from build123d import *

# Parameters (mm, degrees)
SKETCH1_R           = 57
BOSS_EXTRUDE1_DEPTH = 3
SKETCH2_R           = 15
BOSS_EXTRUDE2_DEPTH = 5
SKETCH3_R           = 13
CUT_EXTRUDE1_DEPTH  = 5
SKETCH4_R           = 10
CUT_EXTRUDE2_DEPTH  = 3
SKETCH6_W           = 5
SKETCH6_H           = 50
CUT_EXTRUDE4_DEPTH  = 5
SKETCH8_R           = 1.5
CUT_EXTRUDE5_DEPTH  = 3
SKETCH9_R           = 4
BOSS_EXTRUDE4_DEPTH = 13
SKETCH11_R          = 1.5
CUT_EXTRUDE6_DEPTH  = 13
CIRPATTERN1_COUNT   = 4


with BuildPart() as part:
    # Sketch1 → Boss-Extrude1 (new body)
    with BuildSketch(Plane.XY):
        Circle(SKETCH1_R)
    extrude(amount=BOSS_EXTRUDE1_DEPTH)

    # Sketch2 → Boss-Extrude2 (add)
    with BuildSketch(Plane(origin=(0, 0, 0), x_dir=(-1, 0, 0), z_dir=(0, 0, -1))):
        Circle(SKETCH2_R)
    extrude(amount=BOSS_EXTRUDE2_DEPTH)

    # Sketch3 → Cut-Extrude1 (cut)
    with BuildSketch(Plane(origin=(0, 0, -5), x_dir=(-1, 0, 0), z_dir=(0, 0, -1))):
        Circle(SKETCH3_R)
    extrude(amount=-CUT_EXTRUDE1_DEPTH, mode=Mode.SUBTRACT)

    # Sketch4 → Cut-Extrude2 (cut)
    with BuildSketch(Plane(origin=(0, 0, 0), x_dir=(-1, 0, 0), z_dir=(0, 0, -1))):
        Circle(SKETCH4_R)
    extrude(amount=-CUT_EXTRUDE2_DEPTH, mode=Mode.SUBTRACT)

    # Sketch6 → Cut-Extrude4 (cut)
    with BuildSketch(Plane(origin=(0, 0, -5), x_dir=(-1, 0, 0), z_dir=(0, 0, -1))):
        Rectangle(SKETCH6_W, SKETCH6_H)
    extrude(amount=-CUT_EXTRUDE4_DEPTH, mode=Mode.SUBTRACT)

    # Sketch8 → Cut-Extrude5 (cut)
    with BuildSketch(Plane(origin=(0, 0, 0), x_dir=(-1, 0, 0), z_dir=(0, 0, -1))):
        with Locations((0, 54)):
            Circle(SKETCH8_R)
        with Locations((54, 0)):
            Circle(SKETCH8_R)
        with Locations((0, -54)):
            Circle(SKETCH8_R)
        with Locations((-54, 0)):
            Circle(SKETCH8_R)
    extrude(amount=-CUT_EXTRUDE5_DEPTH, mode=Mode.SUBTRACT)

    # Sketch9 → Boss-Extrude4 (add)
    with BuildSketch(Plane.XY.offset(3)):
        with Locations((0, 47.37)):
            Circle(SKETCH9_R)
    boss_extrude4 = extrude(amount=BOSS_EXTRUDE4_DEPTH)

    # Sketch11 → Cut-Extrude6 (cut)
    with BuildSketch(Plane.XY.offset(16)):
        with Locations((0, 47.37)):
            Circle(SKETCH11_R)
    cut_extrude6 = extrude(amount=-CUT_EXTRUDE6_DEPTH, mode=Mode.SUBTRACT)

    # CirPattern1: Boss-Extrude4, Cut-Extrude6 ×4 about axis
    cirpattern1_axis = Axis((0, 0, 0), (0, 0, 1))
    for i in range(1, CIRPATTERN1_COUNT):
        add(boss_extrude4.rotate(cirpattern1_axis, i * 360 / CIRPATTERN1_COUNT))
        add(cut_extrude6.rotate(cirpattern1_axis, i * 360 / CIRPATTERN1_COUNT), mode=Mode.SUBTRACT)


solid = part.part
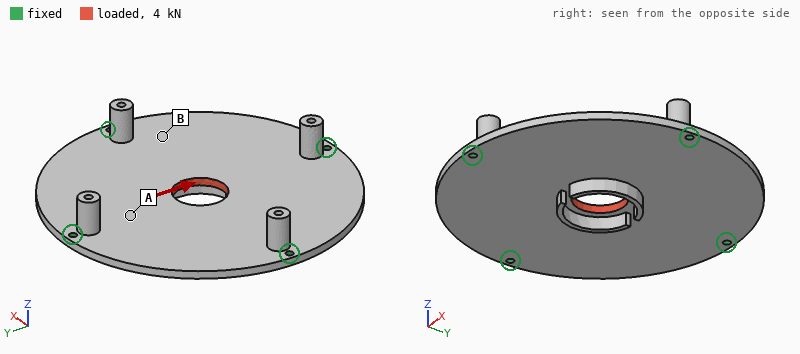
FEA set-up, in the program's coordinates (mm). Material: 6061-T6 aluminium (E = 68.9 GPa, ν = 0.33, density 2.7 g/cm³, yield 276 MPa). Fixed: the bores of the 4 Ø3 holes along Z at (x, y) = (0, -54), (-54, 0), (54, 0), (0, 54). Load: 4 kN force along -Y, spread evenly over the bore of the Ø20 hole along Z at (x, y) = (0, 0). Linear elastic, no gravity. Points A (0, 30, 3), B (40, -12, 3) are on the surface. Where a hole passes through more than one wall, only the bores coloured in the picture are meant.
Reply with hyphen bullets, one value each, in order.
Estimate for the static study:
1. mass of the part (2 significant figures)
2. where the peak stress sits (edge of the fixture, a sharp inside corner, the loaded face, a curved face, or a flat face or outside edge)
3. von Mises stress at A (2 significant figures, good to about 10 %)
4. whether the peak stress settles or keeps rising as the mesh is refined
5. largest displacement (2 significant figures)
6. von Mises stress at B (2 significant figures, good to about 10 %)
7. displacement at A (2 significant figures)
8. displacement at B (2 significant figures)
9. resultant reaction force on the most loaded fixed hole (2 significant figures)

- 88 g
- edge of the fixture
- 21 MPa
- keeps rising
- 16 µm
- 5.6 MPa
- 9.3 µm
- 6.2 µm
- 1.3 kN
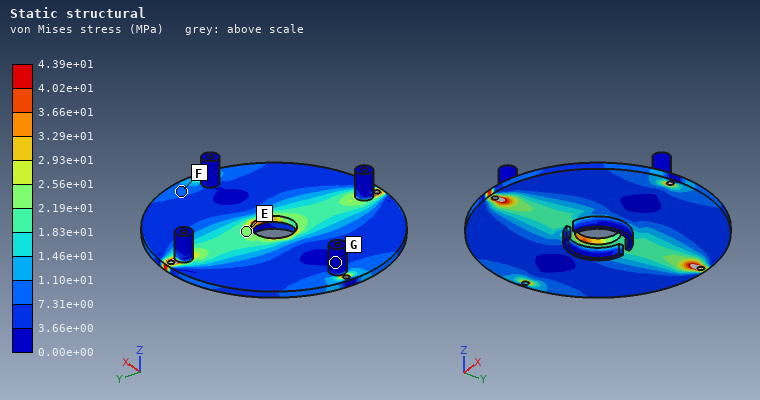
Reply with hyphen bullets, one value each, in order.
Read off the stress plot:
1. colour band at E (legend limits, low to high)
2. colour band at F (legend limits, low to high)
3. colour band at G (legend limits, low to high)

- 2.19e+01 to 2.56e+01 MPa
- 7.31e+00 to 1.10e+01 MPa
- 0.00e+00 to 3.66e+00 MPa
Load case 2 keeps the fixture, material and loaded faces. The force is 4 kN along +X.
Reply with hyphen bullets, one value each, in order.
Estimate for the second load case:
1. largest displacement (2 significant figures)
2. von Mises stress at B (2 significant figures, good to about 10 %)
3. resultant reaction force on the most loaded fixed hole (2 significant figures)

- 16 µm
- 12 MPa
- 1.3 kN
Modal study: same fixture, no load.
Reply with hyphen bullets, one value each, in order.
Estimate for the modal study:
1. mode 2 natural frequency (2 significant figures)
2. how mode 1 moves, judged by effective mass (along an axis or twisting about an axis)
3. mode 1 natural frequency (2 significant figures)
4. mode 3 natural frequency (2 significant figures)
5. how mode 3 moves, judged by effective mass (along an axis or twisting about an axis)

- 2200 Hz
- along Z
- 1800 Hz
- 2400 Hz
- twisting about Y
